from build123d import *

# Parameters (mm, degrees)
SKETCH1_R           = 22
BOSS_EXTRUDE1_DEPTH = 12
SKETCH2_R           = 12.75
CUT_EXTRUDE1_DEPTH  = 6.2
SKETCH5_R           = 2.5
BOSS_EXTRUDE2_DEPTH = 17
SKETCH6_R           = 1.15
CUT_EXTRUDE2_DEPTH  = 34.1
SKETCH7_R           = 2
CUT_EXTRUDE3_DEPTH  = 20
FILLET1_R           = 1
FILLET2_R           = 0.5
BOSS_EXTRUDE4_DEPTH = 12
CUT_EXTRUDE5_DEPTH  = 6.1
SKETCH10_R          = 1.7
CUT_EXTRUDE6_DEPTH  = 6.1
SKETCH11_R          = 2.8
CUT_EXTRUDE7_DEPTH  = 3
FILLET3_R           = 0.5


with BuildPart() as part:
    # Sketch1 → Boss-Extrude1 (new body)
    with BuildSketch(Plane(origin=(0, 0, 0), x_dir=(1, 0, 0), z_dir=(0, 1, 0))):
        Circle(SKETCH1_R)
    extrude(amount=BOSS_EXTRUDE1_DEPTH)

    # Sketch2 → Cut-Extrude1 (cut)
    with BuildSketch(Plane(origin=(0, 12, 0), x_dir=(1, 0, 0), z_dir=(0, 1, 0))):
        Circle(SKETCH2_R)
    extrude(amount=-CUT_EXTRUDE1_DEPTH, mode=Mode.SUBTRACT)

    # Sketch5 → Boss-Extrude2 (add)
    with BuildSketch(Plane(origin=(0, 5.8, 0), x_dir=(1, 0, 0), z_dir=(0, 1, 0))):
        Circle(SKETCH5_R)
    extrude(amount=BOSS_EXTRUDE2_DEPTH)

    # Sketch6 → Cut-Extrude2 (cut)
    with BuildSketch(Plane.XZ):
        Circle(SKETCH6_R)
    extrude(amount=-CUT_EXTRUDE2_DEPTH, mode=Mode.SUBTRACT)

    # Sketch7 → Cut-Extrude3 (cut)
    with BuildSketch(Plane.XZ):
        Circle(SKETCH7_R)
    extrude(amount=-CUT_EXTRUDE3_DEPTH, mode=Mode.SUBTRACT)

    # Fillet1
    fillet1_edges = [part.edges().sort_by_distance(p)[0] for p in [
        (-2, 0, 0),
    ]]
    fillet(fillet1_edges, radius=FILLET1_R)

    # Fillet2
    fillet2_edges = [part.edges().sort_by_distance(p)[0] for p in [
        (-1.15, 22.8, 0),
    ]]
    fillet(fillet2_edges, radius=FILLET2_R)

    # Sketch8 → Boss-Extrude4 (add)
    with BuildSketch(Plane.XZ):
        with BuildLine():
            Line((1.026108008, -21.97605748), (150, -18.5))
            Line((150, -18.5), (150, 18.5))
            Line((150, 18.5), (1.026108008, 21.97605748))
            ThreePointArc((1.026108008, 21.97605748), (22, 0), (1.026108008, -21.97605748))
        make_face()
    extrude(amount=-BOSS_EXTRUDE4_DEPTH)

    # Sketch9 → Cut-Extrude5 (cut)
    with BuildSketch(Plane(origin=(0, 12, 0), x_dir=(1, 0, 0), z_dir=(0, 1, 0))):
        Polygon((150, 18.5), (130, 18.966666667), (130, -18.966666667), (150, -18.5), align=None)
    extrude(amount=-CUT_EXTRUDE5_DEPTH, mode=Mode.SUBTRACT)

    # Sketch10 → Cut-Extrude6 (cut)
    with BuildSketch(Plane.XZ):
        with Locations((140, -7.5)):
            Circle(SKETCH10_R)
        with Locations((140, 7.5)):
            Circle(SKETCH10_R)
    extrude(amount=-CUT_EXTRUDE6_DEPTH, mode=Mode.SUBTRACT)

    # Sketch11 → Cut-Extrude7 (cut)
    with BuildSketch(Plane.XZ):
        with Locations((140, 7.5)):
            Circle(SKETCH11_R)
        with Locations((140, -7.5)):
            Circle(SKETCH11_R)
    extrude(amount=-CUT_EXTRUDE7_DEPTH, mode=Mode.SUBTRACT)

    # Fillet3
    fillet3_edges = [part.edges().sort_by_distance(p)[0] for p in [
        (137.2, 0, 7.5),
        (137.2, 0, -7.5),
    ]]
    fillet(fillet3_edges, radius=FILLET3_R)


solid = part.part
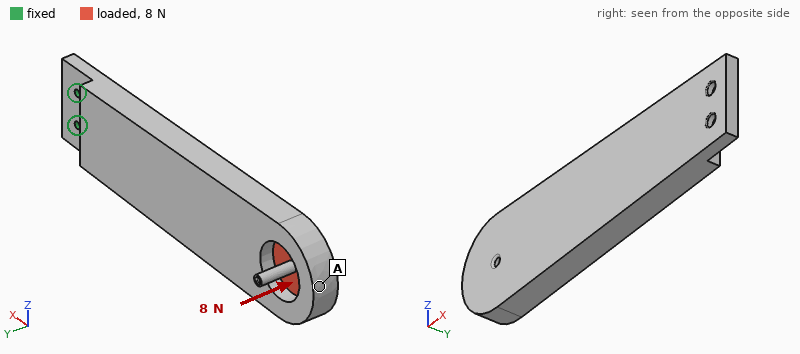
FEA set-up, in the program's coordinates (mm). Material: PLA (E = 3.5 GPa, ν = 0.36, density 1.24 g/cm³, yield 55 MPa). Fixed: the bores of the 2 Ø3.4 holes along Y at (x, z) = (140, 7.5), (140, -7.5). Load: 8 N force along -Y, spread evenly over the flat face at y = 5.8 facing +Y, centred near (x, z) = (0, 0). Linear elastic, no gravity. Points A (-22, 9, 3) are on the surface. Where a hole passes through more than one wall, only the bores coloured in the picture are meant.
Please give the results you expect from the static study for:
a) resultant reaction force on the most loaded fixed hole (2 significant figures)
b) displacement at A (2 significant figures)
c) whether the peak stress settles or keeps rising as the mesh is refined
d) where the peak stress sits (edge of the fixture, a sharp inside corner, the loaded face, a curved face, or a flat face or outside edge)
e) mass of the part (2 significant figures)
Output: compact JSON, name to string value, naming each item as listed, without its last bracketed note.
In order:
{"resultant reaction force on the most loaded fixed hole": "11 N", "displacement at A": "2.1 mm", "whether the peak stress settles or keeps rising as the mesh is refined": "keeps rising", "where the peak stress sits": "edge of the fixture", "mass of the part": "92 g"}
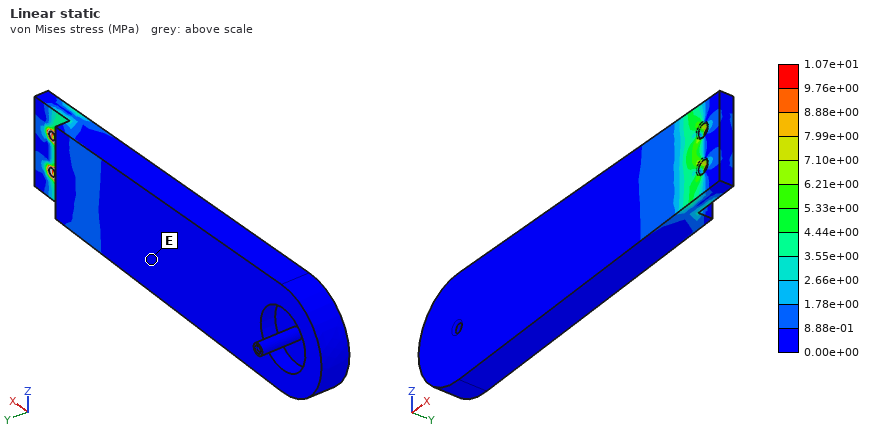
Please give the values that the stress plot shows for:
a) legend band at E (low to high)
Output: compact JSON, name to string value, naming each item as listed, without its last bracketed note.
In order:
{"legend band at E": "0.00e+00 to 8.88e-01 MPa"}
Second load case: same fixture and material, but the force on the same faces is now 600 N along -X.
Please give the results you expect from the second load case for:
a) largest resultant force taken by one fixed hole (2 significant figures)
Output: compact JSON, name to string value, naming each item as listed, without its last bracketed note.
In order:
{"largest resultant force taken by one fixed hole": "300 N"}
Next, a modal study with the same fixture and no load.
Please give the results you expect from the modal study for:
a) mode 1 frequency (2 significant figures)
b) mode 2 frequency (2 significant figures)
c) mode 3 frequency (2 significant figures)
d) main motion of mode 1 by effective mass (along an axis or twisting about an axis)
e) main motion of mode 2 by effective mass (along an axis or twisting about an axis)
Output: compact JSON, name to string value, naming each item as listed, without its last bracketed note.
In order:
{"mode 1 frequency": "55 Hz", "mode 2 frequency": "240 Hz", "mode 3 frequency": "610 Hz", "main motion of mode 1 by effective mass": "along Y", "main motion of mode 2 by effective mass": "along Z"}
